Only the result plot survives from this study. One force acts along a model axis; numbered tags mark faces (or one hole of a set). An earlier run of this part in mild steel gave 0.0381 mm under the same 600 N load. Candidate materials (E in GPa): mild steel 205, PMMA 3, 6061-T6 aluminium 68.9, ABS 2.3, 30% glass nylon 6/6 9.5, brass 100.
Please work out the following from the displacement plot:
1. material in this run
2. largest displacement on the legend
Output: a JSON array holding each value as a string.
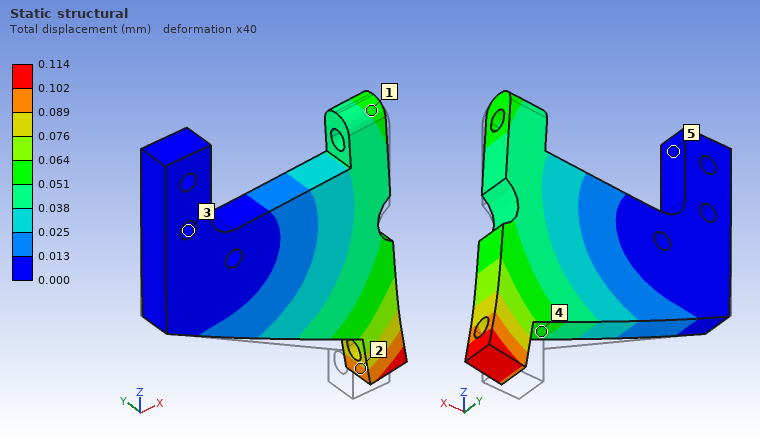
["6061-T6 aluminium", "0.114 mm"]
